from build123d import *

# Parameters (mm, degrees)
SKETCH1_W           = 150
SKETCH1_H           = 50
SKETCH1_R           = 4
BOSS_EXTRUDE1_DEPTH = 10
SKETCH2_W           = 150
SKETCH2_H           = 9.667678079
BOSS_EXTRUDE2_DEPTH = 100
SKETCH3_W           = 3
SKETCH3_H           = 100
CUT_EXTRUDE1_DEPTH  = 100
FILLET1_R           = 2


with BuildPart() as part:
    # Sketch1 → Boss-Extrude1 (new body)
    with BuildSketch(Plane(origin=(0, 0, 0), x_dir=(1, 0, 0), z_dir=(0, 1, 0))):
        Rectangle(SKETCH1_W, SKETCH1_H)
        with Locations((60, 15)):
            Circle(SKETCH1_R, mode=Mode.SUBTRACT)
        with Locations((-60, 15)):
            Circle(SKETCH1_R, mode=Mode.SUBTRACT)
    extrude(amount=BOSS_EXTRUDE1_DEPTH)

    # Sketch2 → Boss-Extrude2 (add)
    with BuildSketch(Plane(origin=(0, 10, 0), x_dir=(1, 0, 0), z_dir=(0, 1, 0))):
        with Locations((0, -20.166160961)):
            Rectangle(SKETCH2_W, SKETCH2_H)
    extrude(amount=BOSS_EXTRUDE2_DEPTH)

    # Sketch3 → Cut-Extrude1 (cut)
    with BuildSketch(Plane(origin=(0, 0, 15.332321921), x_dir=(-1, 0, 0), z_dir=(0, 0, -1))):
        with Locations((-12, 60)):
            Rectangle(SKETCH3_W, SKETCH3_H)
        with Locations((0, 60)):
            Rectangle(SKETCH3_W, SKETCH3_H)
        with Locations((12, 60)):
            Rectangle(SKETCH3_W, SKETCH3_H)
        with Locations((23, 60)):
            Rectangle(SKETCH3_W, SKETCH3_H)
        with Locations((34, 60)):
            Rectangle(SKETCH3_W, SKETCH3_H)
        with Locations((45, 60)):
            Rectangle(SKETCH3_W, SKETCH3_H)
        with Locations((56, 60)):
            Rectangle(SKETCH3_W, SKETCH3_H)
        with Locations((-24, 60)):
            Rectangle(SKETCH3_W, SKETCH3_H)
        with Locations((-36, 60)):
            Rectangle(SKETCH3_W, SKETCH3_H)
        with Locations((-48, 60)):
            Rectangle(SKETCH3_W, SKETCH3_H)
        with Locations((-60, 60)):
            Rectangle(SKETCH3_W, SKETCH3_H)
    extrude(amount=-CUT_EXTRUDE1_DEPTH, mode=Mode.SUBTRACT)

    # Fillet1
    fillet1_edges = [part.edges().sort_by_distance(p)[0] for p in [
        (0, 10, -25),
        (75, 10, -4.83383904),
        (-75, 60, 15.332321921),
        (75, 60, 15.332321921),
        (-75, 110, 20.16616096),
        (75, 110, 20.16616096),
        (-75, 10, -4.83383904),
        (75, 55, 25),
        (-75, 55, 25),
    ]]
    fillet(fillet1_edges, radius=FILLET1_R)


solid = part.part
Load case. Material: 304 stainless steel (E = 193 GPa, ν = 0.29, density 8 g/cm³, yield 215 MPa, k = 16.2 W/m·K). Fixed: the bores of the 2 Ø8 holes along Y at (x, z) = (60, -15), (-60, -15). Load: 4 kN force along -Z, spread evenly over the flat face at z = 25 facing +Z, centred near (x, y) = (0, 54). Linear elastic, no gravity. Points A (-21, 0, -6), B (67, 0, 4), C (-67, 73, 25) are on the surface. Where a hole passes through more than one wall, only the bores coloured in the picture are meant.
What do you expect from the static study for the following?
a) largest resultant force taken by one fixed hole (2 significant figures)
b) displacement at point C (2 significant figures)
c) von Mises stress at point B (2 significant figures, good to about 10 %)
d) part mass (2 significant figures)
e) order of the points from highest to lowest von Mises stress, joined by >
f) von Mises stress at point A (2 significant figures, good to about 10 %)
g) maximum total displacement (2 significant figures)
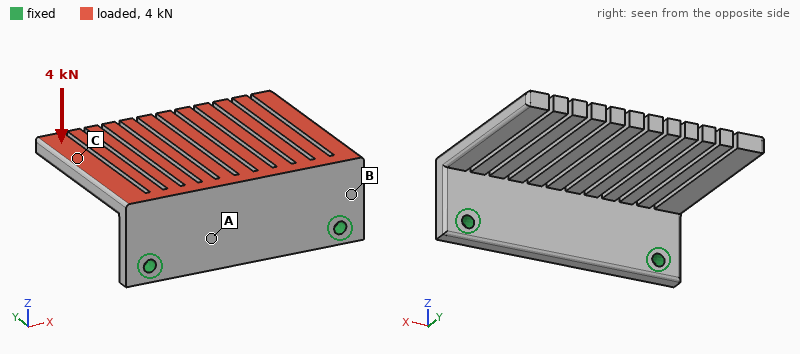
2.2 kN
0.42 mm
110 MPa
1.5 kg
B > A > C
47 MPa
0.80 mm
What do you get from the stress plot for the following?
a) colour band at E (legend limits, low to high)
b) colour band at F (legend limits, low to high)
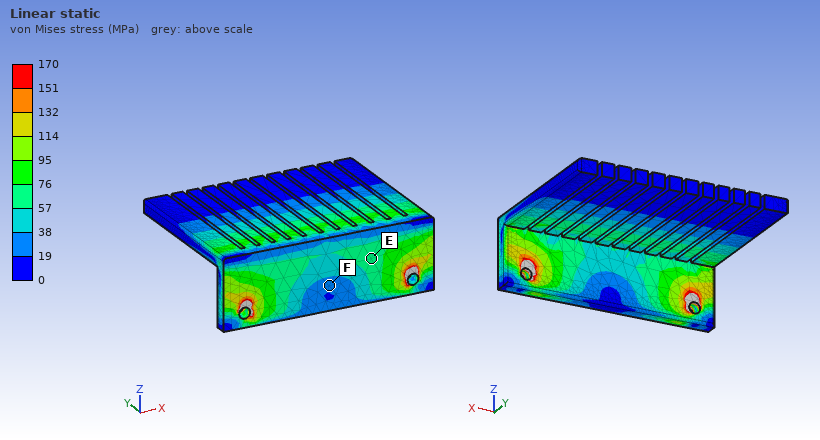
57 to 76 MPa
19 to 38 MPa
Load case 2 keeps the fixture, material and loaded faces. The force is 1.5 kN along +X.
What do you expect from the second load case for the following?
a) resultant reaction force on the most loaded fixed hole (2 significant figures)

1.0 kN
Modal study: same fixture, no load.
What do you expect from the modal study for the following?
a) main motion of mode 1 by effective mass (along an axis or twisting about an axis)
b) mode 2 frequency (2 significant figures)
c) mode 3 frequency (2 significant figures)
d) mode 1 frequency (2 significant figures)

along Z
520 Hz
530 Hz
430 Hz
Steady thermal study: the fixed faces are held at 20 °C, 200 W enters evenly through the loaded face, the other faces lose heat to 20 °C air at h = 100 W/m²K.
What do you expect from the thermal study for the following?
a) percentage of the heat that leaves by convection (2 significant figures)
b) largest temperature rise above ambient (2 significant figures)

95 %
66 K
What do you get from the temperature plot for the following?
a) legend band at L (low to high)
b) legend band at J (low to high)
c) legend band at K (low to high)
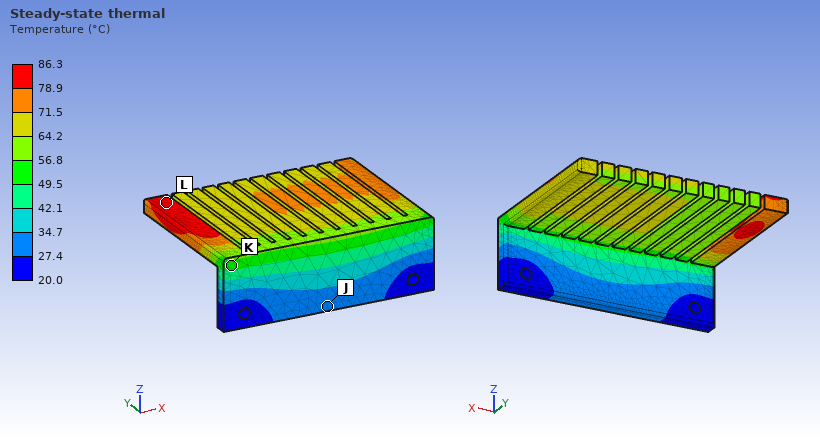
78.9 to 86.3 °C
27.4 to 34.7 °C
49.5 to 56.8 °C
